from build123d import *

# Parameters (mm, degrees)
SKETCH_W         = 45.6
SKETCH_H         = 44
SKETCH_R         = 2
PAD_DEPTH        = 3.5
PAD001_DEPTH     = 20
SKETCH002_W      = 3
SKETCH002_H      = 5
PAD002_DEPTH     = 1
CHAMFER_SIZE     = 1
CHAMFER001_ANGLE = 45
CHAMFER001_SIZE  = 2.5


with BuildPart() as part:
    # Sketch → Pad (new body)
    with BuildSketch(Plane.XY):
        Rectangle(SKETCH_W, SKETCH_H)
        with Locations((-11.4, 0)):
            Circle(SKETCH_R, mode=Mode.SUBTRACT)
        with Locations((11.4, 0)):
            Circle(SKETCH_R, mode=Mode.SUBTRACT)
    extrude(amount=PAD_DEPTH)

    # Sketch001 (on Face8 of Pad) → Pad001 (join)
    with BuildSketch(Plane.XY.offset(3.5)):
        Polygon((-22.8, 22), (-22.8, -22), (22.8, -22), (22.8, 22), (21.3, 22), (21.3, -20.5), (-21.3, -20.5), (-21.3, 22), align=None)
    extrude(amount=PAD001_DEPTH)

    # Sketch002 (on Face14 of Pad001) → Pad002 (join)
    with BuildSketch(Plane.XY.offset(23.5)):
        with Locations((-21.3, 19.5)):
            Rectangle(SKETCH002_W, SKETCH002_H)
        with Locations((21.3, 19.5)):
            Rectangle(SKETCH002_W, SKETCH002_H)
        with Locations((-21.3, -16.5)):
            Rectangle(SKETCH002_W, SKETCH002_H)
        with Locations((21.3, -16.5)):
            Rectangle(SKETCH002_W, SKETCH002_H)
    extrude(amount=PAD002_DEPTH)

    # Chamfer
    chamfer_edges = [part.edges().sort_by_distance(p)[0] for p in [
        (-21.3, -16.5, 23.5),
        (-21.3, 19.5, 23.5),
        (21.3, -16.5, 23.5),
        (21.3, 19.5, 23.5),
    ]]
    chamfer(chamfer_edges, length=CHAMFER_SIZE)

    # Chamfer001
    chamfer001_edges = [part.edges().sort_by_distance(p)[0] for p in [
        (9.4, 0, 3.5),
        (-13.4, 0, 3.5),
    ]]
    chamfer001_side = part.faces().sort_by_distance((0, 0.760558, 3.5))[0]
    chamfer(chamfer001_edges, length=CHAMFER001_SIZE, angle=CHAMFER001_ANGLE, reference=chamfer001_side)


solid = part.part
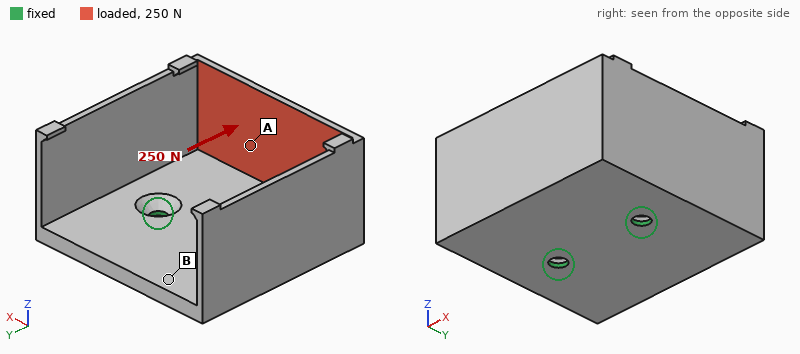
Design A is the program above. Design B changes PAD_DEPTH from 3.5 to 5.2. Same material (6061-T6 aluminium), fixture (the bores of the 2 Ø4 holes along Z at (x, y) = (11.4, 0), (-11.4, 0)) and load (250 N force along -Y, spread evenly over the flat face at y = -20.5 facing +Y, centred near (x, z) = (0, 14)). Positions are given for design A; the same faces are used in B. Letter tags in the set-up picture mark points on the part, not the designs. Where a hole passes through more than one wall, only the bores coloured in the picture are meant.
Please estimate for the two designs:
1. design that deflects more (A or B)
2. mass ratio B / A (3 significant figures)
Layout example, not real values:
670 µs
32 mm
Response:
A
1.28
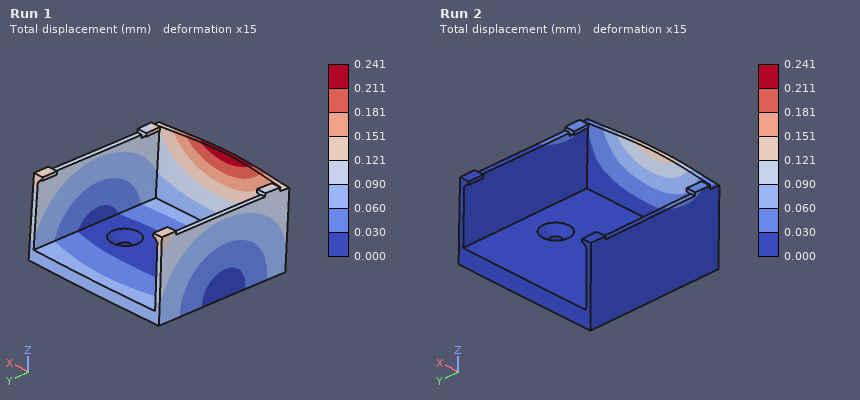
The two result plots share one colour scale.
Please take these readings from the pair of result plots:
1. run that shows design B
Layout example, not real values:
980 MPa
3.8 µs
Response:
Run 2
